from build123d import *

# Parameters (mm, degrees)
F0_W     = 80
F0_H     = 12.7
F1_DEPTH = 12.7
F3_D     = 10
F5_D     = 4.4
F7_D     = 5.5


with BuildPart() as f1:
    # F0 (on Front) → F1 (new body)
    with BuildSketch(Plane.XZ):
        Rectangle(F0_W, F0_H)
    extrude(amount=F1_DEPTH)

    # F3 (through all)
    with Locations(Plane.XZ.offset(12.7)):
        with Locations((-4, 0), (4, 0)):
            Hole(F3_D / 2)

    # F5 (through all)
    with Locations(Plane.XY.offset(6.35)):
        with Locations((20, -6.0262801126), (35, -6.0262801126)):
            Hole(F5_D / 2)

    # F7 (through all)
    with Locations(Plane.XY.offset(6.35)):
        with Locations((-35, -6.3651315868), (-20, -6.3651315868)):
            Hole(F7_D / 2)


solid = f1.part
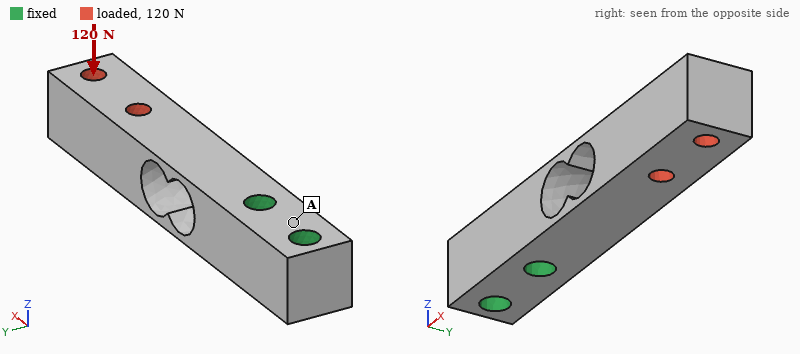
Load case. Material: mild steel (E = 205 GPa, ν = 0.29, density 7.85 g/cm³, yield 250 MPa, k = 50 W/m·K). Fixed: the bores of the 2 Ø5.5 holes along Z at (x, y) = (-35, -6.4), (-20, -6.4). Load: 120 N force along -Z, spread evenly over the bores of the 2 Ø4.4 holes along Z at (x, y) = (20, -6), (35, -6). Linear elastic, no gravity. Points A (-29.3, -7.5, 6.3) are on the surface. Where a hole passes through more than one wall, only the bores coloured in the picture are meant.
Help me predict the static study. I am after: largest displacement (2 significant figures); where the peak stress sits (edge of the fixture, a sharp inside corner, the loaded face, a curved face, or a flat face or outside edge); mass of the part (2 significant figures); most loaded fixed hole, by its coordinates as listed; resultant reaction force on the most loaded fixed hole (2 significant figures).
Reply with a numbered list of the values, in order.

1. 37 µm
2. a curved face
3. 79 g
4. (-20, -6.4)
5. 150 N
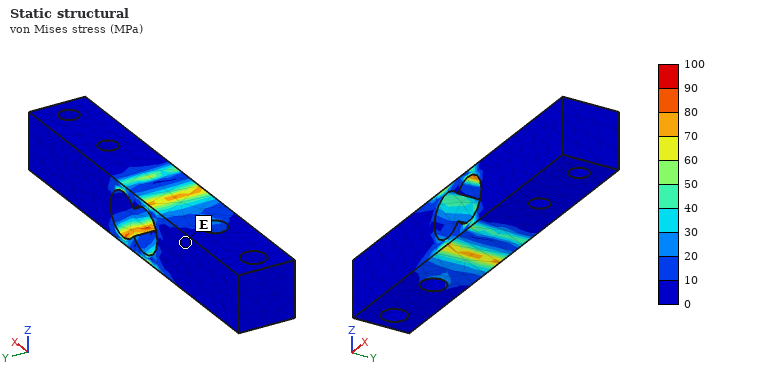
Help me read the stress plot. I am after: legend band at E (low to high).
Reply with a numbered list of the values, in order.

1. 0 to 10 MPa
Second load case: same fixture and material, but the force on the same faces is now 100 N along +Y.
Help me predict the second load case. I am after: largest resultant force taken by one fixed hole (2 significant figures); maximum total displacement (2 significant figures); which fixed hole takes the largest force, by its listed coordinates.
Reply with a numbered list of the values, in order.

1. 190 N
2. 29 µm
3. (-20, -6.4)
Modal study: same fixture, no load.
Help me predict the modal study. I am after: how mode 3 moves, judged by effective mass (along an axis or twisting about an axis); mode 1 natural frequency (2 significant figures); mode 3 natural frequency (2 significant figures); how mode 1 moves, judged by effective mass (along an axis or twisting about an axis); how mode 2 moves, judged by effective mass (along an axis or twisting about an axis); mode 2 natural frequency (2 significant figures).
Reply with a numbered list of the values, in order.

1. twisting about X
2. 1600 Hz
3. 7000 Hz
4. along Z
5. along Y
6. 1900 Hz
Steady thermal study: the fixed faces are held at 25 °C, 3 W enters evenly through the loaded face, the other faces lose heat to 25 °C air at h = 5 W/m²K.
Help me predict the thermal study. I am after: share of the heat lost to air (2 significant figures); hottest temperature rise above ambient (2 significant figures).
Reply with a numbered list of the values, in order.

1. 11 %
2. 32 K
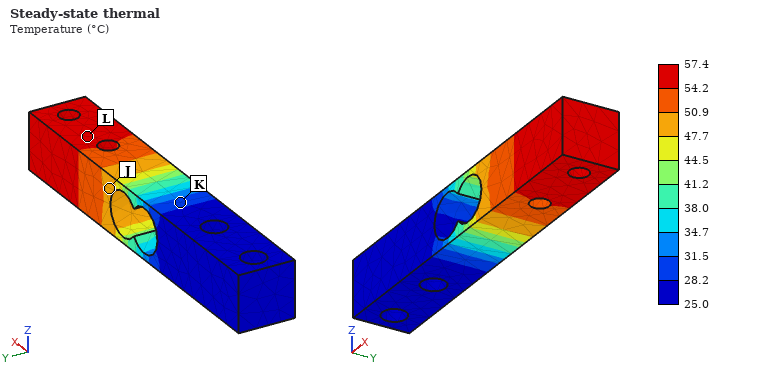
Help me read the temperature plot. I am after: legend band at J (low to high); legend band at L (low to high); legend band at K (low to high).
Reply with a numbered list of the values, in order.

1. 47.7 to 50.9 °C
2. 54.2 to 57.4 °C
3. 28.2 to 31.5 °C
